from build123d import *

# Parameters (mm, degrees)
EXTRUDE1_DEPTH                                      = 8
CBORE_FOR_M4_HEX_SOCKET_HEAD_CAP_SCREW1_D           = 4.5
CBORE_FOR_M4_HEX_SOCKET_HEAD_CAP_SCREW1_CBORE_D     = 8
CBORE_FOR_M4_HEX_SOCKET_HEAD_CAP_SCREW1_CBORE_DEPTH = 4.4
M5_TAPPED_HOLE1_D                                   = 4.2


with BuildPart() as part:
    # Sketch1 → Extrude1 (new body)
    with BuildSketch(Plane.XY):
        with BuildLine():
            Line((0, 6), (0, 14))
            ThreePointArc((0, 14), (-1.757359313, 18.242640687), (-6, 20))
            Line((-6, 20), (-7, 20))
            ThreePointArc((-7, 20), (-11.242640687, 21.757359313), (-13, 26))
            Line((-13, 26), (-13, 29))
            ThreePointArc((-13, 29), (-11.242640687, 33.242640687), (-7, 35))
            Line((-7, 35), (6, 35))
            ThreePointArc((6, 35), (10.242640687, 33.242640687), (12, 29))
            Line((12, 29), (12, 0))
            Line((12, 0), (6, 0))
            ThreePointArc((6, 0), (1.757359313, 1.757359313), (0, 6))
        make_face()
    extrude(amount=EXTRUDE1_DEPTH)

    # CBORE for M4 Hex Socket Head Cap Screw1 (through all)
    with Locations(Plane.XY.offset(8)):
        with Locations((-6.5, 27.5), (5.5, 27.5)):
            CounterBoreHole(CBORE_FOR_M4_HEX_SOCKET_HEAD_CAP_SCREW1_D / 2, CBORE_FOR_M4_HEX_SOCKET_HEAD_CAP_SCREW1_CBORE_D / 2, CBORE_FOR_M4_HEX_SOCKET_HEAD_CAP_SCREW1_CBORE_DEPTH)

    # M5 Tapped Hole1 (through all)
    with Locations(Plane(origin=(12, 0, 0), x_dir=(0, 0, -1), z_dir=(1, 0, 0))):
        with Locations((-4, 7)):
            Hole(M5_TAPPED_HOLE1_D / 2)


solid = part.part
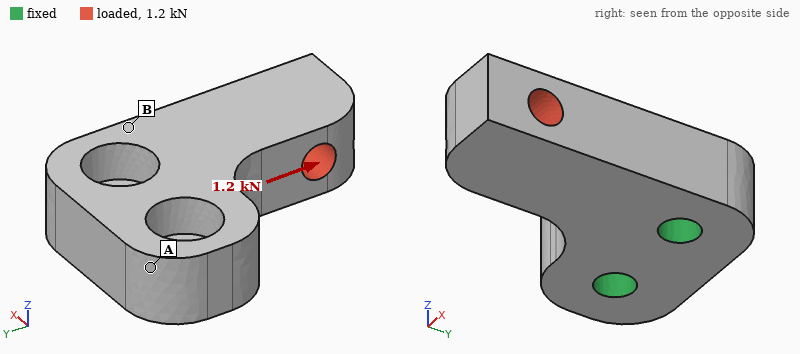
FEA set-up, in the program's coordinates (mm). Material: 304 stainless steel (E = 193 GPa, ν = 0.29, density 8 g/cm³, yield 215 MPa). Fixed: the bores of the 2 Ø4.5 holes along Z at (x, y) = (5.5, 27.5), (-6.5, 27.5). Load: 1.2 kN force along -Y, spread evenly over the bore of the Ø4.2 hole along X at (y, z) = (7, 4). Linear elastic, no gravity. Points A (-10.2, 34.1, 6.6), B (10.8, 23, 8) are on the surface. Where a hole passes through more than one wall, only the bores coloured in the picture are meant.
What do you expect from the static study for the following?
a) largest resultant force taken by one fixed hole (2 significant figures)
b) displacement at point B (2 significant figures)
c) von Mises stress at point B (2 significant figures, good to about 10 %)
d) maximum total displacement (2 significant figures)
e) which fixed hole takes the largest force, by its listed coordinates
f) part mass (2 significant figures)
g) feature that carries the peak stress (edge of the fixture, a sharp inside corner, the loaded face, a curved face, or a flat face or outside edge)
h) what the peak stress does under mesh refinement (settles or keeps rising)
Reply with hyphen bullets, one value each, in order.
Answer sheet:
- 1.1 kN
- 2.6 µm
- 18 MPa
- 7.7 µm
- (5.5, 27.5)
- 32 g
- edge of the fixture
- keeps rising
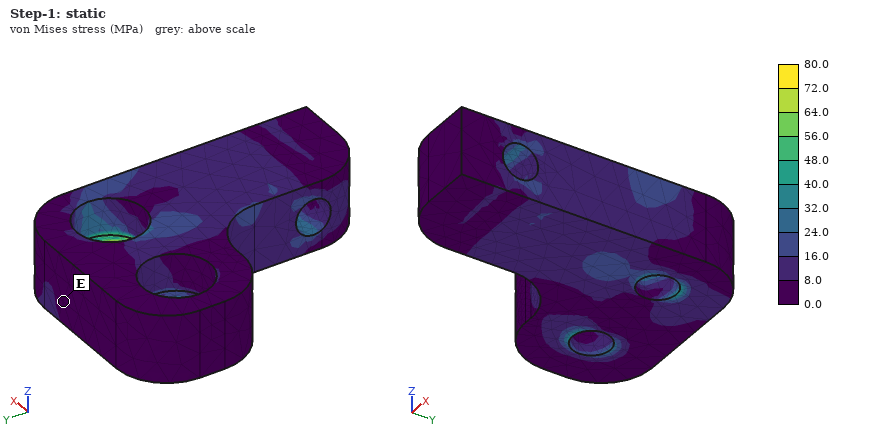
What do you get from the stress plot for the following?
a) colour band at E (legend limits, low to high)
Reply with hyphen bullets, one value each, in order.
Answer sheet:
- 0.0 to 8.0 MPa
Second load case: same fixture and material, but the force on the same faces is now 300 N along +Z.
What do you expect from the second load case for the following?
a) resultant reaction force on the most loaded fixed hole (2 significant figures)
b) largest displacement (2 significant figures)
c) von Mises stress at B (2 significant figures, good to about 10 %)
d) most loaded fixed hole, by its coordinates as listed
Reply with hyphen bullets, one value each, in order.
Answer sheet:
- 300 N
- 23 µm
- 37 MPa
- (5.5, 27.5)
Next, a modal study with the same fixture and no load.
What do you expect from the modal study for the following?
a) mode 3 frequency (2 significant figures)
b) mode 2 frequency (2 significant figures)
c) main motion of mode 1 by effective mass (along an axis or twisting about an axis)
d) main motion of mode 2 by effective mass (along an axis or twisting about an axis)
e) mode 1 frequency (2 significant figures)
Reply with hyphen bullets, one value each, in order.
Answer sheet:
- 27 kHz
- 14 kHz
- along Z
- along X
- 6900 Hz
